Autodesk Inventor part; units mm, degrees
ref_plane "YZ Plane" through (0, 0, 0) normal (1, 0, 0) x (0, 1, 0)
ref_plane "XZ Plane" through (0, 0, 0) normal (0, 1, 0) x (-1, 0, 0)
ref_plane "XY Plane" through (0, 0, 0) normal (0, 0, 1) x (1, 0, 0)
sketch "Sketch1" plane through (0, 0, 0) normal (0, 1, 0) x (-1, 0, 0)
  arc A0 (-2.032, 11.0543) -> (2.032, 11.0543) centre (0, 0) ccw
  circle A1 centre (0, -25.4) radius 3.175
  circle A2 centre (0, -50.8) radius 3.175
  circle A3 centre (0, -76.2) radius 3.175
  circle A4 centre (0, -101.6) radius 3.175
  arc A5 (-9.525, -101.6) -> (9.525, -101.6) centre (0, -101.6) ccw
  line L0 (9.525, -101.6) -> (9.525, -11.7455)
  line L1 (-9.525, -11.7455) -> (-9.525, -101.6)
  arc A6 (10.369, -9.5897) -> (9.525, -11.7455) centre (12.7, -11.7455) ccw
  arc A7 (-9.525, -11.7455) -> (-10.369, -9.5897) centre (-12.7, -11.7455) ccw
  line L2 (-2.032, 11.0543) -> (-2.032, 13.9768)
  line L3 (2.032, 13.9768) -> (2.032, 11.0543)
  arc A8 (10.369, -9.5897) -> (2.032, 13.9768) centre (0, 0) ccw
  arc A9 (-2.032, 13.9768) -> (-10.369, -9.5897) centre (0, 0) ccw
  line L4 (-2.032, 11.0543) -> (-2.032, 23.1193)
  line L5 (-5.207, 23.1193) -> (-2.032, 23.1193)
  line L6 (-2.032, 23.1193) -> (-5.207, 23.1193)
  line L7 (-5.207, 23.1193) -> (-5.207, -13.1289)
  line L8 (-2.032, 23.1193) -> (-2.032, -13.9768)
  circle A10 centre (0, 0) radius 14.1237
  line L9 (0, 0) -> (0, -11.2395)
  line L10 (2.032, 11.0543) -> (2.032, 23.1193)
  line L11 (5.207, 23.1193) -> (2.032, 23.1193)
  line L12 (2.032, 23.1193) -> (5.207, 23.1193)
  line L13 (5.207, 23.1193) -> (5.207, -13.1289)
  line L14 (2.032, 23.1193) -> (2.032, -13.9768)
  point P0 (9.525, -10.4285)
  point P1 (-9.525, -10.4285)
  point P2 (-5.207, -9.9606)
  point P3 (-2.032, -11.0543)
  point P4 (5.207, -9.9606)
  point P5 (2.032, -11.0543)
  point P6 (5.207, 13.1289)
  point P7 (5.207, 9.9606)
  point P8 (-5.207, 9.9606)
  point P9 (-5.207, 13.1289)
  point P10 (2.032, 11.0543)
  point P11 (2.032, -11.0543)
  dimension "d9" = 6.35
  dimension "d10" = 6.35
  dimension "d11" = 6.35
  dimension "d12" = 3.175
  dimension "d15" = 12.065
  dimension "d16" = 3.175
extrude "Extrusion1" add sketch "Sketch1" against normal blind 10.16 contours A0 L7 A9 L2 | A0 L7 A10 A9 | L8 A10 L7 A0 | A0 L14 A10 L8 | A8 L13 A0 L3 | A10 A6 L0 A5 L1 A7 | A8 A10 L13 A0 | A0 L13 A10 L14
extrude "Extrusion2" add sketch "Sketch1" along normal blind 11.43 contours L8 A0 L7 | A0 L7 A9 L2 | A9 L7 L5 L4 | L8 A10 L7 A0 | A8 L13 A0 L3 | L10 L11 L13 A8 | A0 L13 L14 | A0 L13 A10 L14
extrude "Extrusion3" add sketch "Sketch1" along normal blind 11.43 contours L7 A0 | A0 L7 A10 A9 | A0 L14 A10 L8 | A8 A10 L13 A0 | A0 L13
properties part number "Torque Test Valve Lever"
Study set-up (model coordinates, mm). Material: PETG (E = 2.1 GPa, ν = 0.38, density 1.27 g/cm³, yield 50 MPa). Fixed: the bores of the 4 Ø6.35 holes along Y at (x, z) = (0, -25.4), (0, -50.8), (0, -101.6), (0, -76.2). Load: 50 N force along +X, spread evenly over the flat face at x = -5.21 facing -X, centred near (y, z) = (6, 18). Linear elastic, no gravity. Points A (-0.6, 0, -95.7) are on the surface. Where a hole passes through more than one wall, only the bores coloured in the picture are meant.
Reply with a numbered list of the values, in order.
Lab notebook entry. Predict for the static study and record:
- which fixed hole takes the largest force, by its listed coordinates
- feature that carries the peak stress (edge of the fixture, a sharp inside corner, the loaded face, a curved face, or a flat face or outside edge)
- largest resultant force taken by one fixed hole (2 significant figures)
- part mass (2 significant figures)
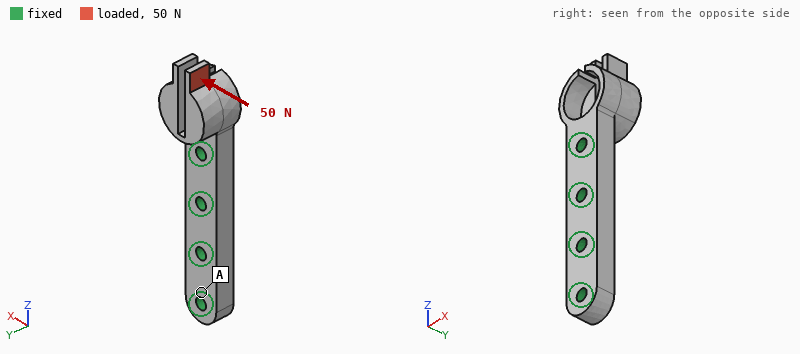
1. (0, -25.4)
2. a curved face
3. 89 N
4. 33 g
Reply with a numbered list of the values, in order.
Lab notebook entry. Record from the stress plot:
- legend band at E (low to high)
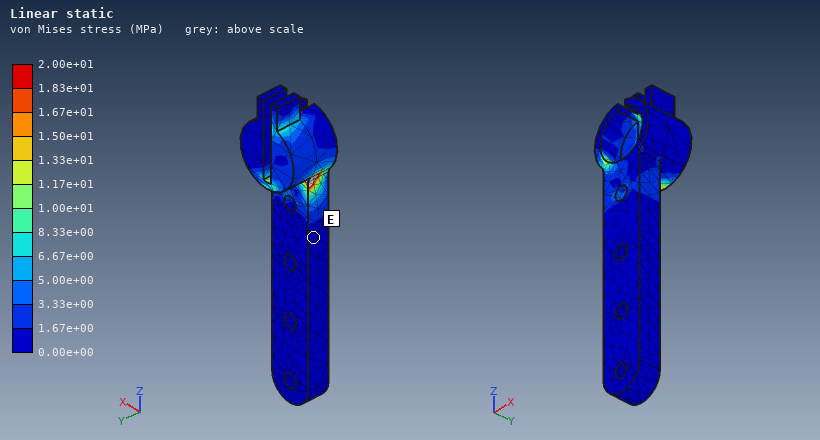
1. 0.00e+00 to 1.67e+00 MPa
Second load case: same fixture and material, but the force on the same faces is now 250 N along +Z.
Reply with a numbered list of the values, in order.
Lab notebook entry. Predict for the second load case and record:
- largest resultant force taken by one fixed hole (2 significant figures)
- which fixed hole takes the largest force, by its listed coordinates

1. 230 N
2. (0, -25.4)
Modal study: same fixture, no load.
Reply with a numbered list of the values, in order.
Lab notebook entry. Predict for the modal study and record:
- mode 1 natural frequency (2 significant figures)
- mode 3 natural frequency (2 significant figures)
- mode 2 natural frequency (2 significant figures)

1. 710 Hz
2. 990 Hz
3. 730 Hz
